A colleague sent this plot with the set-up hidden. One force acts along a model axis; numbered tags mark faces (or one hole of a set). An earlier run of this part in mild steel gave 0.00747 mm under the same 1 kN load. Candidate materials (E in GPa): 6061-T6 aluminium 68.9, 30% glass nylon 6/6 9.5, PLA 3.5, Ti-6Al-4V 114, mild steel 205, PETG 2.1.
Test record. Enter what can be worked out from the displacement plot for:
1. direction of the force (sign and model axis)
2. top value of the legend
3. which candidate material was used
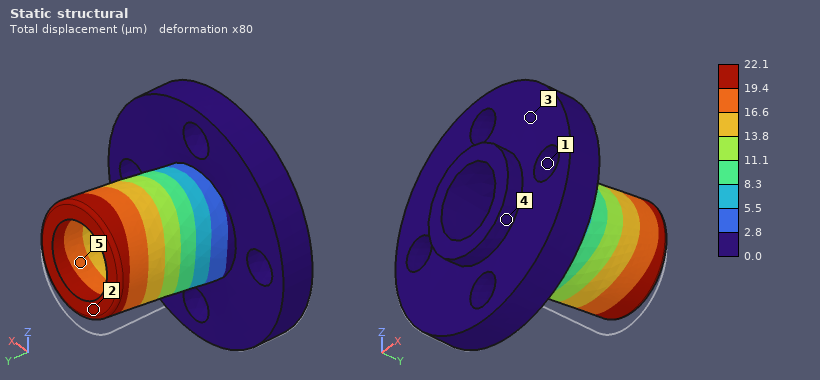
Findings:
+Z
22.1 µm
6061-T6 aluminium
